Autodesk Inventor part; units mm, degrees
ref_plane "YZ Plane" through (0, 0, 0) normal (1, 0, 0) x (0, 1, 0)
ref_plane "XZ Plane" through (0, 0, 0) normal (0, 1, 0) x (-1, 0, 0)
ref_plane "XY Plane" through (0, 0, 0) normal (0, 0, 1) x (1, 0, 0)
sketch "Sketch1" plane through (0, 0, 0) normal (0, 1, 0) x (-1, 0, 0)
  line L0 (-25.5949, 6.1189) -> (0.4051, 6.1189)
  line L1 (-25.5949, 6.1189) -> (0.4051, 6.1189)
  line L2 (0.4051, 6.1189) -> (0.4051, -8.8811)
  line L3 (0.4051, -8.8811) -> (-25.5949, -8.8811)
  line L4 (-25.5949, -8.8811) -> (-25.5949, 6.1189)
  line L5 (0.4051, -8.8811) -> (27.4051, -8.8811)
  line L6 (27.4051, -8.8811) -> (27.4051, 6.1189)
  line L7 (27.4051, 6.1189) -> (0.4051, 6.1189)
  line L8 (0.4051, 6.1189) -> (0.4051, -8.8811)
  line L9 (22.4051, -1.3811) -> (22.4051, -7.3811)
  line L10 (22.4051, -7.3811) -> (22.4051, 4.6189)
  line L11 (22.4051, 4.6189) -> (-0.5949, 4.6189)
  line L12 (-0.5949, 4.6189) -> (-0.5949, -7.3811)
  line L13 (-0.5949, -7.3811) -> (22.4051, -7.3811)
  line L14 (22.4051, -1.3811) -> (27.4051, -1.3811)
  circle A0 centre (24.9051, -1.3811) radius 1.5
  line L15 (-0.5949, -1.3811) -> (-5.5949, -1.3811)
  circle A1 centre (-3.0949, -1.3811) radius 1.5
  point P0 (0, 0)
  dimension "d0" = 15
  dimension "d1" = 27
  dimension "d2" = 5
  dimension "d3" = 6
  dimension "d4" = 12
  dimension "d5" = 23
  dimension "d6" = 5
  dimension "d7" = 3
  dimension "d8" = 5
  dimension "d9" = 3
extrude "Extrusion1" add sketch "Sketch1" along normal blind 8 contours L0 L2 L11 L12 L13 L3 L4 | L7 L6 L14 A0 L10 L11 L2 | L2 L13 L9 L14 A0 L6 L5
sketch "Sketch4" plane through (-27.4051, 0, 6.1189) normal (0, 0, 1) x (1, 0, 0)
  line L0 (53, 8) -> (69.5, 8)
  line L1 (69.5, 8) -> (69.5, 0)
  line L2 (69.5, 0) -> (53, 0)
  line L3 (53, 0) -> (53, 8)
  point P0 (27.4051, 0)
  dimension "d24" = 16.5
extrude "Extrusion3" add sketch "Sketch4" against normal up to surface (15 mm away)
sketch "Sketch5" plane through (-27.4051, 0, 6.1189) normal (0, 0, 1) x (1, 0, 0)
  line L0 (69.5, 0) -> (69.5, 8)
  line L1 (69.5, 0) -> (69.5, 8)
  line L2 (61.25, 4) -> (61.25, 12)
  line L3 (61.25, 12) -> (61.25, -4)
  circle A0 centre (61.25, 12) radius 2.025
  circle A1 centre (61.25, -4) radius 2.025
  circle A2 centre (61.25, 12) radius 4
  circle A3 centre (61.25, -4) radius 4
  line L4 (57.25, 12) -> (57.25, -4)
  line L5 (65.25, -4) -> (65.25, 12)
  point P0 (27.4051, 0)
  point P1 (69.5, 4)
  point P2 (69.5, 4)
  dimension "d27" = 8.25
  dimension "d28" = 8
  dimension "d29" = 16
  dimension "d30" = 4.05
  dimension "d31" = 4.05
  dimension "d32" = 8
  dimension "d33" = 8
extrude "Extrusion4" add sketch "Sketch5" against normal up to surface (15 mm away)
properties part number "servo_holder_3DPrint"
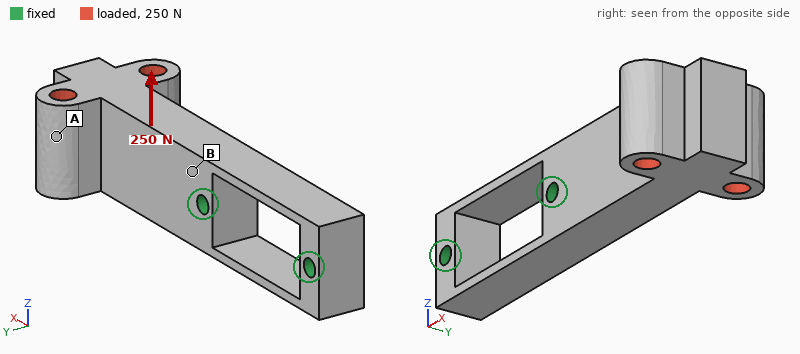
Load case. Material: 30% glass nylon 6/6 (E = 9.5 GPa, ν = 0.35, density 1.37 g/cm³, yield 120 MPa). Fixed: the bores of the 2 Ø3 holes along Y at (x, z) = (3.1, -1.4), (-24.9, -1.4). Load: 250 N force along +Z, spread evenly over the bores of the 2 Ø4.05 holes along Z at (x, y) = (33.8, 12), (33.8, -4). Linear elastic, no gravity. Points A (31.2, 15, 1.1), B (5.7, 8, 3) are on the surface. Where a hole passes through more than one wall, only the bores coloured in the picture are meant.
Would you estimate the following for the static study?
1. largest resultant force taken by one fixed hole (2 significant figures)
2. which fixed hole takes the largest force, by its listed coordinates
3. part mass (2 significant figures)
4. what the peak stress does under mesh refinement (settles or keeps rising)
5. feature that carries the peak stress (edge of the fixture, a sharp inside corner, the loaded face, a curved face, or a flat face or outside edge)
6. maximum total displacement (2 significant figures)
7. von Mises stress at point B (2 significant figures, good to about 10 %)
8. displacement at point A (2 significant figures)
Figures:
260 N
(3.1, -1.4)
10 g
keeps rising
edge of the fixture
0.47 mm
17 MPa
0.32 mm
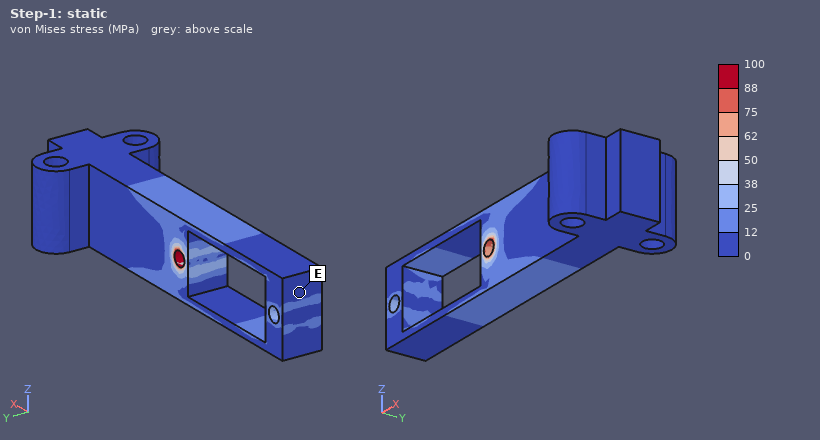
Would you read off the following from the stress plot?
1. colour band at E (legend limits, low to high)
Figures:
0 to 12 MPa
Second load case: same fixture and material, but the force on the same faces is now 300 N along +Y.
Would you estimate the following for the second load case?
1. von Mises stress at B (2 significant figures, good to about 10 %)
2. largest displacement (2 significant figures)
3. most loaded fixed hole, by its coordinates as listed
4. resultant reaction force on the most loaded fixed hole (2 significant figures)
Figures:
36 MPa
0.79 mm
(3.1, -1.4)
340 N
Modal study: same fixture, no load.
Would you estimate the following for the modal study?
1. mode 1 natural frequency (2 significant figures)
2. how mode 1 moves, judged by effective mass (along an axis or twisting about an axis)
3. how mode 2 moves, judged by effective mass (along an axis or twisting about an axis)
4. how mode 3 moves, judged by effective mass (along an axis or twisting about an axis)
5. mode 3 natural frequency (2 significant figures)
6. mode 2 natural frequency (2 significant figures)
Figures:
1600 Hz
along Y
along Z
twisting about X
4800 Hz
1800 Hz
